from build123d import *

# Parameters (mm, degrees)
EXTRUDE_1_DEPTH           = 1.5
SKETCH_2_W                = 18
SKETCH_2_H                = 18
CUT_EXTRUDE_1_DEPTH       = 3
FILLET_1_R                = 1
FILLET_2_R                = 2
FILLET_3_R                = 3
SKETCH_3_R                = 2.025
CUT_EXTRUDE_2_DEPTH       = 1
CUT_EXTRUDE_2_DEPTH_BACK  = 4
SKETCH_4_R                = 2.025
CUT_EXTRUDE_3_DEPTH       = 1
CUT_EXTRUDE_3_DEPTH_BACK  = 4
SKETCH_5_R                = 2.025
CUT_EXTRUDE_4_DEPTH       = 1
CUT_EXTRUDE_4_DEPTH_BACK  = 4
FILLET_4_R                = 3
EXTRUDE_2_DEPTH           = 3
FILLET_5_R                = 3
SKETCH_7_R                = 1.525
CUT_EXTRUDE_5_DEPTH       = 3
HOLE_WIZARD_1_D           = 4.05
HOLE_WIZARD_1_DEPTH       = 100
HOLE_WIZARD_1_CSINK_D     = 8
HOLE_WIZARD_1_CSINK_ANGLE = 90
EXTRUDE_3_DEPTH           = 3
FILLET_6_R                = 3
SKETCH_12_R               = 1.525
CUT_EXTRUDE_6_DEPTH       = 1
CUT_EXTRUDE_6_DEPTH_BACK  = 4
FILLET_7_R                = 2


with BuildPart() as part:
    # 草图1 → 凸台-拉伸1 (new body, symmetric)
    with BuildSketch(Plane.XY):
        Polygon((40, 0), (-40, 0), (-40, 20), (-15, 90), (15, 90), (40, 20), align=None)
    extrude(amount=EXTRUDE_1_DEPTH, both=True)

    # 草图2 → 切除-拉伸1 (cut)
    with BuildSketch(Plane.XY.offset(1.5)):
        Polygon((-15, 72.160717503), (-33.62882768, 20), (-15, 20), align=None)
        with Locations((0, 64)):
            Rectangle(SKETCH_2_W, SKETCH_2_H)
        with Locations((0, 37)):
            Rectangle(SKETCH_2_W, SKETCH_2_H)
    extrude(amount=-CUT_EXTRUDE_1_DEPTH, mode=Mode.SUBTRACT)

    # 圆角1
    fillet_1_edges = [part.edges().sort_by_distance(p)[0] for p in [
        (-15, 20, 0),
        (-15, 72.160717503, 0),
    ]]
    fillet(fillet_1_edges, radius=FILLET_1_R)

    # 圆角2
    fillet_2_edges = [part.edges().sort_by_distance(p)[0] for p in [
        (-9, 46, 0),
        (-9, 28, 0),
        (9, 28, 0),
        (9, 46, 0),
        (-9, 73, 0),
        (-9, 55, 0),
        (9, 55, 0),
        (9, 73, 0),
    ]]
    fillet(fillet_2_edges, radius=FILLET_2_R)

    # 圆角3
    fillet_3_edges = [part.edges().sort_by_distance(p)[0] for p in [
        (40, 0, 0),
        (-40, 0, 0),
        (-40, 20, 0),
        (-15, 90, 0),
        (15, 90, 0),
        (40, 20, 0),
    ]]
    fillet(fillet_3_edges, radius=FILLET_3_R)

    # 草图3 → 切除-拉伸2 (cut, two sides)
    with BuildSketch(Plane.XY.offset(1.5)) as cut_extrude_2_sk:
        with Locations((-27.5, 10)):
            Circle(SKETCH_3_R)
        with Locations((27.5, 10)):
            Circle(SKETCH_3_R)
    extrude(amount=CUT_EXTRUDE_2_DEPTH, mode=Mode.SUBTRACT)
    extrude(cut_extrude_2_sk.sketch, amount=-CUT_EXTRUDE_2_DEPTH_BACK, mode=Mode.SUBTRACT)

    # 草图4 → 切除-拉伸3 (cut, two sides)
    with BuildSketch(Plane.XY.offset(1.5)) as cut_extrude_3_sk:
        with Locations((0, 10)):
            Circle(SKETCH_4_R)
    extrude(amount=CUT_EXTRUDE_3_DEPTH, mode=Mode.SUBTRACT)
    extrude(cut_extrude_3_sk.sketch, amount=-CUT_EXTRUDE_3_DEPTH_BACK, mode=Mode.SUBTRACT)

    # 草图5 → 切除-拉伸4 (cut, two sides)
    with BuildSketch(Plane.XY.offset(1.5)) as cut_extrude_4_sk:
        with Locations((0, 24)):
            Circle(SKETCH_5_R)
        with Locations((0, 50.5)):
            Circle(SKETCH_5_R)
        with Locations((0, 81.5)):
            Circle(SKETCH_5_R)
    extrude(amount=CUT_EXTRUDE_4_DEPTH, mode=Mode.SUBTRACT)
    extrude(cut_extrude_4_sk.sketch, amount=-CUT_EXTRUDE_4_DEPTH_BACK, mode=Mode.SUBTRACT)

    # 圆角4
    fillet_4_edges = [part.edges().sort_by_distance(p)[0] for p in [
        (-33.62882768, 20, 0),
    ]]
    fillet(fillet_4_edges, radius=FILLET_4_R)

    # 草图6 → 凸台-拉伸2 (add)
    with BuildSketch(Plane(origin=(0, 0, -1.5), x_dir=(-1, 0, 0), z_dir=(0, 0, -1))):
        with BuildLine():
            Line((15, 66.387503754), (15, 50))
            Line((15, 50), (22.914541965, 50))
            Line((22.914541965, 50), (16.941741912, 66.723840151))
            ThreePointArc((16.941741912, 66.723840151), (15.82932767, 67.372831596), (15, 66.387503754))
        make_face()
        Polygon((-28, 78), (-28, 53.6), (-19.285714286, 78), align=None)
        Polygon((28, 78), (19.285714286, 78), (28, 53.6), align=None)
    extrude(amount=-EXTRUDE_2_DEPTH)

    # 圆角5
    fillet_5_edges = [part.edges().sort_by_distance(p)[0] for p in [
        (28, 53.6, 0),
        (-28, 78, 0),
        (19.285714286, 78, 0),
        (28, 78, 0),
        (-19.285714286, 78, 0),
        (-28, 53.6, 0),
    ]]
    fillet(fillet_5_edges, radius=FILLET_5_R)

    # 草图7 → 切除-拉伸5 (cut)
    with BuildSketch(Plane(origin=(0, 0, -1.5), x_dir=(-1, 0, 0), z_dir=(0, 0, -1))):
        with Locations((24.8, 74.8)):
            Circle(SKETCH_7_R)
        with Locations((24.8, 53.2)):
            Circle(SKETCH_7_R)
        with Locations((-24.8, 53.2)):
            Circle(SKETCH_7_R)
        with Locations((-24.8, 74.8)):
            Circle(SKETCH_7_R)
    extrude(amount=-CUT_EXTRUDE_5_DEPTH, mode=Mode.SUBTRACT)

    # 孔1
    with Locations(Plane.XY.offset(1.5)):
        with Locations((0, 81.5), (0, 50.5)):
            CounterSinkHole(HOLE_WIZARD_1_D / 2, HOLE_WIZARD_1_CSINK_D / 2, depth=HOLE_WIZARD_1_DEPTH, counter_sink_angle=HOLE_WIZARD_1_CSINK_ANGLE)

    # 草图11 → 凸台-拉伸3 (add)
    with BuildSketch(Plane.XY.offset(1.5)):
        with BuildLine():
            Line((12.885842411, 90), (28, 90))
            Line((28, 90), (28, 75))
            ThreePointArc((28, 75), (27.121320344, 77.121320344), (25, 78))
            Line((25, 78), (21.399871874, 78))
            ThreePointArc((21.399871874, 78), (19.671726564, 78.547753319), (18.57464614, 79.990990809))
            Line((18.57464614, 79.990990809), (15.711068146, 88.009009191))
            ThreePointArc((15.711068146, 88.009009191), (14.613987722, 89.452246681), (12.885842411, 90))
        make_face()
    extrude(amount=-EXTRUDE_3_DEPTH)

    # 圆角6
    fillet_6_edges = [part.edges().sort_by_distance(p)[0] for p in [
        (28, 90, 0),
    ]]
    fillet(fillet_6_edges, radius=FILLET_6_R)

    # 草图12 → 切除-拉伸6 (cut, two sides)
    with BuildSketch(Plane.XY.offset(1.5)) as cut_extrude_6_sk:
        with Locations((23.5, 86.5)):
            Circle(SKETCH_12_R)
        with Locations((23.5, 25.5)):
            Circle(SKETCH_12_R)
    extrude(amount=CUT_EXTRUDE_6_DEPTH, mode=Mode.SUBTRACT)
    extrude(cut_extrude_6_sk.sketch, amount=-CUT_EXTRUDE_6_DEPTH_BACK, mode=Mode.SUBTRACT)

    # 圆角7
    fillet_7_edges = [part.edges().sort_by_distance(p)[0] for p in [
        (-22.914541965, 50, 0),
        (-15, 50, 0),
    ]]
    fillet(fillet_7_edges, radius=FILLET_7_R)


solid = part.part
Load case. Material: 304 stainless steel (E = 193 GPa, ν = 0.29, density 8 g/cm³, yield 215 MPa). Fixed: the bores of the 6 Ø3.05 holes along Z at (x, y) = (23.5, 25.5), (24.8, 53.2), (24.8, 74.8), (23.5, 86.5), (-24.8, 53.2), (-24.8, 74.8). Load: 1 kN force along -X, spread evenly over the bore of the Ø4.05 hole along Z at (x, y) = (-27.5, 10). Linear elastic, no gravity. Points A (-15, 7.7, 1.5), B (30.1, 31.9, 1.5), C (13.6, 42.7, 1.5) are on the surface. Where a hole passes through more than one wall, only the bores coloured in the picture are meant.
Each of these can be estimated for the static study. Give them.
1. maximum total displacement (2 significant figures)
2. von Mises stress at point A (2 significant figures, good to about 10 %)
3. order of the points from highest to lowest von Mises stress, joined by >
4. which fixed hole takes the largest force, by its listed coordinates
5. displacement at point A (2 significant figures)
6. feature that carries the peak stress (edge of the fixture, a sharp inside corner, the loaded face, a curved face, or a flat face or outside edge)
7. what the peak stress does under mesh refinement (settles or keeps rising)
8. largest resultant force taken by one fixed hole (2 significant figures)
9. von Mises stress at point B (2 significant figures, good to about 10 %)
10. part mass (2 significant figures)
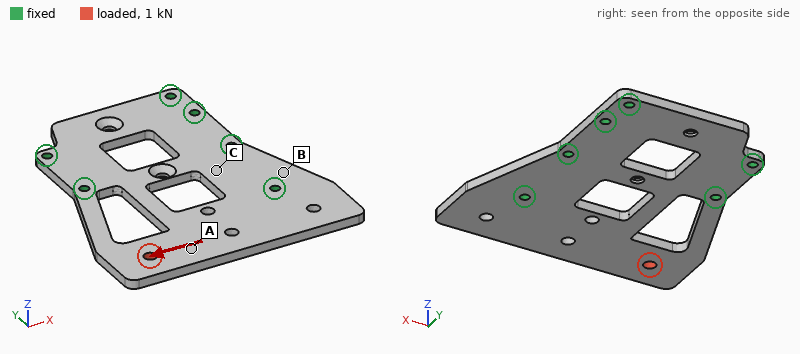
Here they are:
7.9 µm
15 MPa
A > B > C
(23.5, 25.5)
6.3 µm
edge of the fixture
keeps rising
1.1 kN
7.9 MPa
110 g
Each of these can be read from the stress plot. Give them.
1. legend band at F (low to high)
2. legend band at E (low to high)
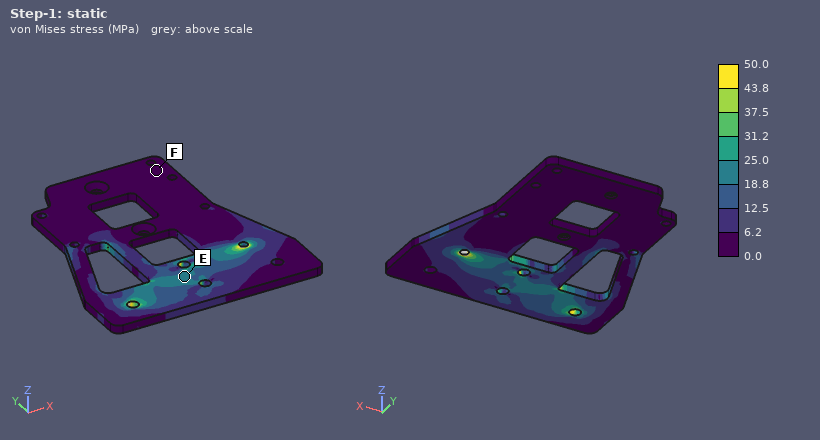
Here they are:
0.0 to 6.2 MPa
18.8 to 25.0 MPa
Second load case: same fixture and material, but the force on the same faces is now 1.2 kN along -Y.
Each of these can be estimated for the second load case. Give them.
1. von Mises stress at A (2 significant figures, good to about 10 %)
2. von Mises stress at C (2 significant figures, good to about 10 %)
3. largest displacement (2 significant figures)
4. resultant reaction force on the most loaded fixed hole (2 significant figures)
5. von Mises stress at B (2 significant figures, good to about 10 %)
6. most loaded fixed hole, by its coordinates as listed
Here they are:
16 MPa
7.4 MPa
12 µm
910 N
6.1 MPa
(-24.8, 53.2)
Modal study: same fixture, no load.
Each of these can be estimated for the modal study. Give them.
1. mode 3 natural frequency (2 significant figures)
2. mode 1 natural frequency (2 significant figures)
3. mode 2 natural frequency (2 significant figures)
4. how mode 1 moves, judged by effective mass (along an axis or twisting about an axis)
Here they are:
3900 Hz
950 Hz
2800 Hz
along Z
